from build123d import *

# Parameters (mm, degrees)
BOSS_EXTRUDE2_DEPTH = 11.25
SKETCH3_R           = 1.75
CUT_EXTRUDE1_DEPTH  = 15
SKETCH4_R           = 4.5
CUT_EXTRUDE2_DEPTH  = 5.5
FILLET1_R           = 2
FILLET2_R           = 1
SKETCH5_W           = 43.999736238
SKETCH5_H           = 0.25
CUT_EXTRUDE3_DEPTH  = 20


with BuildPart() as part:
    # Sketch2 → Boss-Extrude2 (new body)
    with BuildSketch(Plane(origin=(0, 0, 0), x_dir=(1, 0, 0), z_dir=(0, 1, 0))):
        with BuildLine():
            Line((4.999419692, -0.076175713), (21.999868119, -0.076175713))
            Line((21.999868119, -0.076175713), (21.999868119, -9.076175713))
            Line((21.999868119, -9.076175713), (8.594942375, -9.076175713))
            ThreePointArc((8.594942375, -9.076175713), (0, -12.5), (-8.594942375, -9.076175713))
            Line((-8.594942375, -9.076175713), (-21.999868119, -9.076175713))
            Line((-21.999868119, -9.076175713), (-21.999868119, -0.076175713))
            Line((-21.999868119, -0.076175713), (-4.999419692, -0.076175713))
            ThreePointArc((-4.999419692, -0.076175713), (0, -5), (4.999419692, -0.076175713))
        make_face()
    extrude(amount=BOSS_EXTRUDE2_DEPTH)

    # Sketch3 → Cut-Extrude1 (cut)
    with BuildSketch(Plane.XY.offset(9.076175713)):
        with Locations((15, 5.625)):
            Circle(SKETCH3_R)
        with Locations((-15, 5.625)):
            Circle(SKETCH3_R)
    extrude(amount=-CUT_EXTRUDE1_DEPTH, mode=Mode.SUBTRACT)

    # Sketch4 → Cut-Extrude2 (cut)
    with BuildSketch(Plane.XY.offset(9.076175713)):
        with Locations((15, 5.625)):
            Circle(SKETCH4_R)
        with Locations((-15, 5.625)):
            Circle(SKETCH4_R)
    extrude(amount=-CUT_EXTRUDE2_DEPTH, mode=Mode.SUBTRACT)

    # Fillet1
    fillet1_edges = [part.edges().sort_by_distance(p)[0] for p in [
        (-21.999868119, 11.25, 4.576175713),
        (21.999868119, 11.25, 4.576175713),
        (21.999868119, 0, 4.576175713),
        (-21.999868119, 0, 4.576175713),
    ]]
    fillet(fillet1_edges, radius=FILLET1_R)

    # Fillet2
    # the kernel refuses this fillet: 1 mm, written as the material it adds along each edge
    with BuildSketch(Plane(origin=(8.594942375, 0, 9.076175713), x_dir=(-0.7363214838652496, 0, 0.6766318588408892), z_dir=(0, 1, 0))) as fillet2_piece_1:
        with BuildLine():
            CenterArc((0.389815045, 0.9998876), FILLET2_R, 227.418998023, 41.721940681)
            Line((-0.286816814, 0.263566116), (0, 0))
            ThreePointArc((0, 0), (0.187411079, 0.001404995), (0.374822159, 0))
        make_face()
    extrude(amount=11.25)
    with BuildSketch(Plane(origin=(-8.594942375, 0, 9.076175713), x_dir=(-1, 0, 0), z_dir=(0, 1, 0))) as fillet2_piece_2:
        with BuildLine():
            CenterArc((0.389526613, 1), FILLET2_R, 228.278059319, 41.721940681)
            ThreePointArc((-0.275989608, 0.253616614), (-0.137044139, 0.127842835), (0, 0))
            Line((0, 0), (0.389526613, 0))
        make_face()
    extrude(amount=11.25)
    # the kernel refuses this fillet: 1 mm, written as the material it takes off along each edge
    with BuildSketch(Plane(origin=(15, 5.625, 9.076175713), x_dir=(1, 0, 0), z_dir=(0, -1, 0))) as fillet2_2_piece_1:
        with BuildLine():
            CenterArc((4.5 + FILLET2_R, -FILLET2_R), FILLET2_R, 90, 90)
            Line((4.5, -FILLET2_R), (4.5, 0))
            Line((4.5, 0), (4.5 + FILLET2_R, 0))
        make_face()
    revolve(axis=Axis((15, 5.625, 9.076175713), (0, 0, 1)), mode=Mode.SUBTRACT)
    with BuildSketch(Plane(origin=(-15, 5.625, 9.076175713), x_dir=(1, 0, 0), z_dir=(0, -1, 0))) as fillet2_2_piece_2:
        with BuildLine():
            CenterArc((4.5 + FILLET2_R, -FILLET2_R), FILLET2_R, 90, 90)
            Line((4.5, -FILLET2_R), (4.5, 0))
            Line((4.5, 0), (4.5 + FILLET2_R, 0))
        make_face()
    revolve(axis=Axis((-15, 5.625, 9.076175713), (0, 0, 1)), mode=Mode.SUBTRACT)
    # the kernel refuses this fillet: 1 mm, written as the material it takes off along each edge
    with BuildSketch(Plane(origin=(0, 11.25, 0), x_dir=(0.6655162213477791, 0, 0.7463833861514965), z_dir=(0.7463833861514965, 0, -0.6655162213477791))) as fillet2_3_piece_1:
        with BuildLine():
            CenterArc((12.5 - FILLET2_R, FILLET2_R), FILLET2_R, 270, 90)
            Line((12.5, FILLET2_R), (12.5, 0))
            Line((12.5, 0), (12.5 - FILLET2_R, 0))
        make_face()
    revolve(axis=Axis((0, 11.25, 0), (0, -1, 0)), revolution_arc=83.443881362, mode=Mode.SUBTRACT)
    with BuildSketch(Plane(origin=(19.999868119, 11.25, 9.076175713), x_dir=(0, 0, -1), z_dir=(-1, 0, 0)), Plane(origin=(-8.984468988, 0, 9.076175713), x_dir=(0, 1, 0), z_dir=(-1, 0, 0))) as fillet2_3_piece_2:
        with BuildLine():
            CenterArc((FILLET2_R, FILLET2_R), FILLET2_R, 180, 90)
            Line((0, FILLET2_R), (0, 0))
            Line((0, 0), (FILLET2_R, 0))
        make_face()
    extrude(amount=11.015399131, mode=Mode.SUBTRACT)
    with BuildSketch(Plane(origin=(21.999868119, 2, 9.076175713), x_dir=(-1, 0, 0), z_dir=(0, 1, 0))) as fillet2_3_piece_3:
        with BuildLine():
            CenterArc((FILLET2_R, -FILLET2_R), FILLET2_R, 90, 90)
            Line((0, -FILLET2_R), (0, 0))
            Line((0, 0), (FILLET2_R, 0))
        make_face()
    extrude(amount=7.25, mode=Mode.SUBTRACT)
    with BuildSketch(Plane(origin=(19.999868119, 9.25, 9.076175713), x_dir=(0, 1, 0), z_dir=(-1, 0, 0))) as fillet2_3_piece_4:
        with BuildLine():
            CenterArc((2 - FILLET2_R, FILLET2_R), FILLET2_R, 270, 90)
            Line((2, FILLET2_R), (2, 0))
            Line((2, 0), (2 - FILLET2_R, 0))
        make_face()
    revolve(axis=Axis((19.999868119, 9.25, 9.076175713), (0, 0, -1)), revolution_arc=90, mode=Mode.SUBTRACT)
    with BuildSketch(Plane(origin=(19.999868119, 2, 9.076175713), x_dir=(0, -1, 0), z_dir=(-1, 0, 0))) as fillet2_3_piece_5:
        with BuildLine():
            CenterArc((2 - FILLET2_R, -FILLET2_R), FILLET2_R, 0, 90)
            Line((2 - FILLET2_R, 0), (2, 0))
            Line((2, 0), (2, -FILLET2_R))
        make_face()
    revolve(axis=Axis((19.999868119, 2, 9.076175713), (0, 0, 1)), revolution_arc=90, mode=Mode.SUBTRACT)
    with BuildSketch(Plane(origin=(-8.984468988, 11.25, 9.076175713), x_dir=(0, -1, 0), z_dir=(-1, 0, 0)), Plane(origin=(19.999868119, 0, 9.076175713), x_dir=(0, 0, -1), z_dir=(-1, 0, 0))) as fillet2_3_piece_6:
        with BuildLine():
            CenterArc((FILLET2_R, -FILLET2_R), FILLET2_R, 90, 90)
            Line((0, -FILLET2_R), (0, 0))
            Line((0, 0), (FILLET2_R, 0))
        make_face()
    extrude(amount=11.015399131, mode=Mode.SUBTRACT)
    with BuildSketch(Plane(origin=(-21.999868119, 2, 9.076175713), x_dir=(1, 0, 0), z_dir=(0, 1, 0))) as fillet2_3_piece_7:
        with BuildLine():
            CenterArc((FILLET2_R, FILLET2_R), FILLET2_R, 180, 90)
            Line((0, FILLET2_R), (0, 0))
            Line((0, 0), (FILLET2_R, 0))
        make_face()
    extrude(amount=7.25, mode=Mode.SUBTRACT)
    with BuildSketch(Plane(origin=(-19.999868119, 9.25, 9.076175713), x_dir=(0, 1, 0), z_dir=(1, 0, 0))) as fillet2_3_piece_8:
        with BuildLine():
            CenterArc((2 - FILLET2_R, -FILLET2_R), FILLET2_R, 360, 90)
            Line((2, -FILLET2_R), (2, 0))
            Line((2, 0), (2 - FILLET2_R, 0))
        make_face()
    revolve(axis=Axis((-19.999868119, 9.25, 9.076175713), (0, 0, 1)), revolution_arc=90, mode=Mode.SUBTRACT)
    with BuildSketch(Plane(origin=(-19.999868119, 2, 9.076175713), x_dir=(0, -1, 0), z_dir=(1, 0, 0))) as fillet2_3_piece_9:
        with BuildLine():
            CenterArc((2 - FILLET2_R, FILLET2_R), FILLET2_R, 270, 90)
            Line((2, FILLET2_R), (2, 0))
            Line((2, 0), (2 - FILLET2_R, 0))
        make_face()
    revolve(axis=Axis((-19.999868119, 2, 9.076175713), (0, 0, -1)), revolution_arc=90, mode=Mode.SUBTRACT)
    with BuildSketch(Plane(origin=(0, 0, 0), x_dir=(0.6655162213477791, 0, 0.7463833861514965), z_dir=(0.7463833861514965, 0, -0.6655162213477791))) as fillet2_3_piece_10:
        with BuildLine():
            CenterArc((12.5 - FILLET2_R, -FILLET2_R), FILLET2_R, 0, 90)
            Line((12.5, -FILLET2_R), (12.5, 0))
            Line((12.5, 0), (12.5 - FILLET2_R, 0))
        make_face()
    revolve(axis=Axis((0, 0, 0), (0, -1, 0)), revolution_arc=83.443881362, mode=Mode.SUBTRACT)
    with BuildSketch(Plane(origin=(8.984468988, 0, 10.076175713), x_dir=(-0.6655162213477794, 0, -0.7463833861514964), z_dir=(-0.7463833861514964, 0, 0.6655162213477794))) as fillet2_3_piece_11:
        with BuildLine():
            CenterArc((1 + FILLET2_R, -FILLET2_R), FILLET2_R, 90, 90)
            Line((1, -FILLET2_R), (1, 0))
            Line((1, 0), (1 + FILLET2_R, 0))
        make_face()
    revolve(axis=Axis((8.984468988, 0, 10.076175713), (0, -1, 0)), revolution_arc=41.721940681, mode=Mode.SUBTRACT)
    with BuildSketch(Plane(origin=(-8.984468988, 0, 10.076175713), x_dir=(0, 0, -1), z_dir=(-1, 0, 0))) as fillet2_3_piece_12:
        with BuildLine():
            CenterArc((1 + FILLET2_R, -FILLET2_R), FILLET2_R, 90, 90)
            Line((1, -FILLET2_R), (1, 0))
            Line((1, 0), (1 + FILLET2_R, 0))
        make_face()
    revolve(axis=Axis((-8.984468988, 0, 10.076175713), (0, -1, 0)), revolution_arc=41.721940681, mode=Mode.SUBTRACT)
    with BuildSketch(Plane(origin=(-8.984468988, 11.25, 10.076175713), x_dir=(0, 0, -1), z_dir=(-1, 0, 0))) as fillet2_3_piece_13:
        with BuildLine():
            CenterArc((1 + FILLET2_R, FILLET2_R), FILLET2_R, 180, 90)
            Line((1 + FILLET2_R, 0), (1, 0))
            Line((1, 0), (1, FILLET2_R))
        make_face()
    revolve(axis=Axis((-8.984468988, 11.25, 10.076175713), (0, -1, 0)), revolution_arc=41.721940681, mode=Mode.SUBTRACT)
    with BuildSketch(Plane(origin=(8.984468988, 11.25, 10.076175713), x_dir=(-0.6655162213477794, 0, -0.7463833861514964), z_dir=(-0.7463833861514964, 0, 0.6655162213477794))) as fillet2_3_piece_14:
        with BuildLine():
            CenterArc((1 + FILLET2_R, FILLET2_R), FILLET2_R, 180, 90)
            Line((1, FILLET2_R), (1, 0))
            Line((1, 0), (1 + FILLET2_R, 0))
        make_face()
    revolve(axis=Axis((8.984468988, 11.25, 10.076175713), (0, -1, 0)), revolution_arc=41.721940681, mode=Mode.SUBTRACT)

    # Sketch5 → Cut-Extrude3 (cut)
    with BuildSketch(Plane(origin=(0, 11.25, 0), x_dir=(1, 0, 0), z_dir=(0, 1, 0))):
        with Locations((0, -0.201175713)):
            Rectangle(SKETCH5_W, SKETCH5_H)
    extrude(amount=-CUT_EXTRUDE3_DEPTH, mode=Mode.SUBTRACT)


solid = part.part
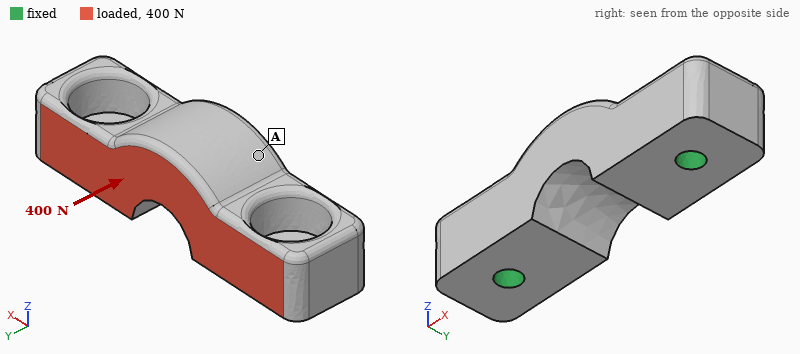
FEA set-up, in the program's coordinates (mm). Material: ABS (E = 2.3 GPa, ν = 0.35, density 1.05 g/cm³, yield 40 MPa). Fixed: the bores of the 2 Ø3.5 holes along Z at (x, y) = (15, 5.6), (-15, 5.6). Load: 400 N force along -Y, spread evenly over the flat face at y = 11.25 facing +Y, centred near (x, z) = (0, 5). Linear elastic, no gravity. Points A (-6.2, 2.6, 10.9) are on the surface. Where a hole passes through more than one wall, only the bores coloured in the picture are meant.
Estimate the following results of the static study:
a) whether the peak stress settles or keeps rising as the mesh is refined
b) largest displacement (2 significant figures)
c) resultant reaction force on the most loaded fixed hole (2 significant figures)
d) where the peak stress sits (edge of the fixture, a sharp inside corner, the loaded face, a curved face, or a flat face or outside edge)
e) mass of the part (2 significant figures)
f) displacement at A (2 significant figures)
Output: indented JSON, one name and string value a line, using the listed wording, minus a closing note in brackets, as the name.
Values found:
{
  "whether the peak stress settles or keeps rising as the mesh is refined": "keeps rising",
  "largest displacement": "0.20 mm",
  "resultant reaction force on the most loaded fixed hole": "200 N",
  "where the peak stress sits": "edge of the fixture",
  "mass of the part": "3.7 g",
  "displacement at A": "0.17 mm"
}
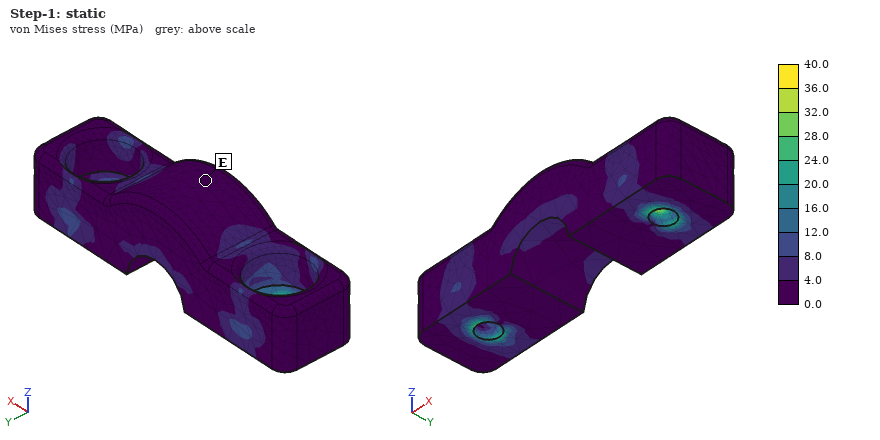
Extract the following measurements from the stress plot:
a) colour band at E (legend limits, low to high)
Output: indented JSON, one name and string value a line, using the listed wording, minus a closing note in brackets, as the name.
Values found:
{
  "colour band at E": "0.0 to 4.0 MPa"
}
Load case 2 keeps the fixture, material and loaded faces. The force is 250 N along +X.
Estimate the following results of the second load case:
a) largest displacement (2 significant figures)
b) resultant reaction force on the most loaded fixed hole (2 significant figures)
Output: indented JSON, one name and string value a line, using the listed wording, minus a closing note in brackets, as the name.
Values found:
{
  "largest displacement": "29 µm",
  "resultant reaction force on the most loaded fixed hole": "130 N"
}
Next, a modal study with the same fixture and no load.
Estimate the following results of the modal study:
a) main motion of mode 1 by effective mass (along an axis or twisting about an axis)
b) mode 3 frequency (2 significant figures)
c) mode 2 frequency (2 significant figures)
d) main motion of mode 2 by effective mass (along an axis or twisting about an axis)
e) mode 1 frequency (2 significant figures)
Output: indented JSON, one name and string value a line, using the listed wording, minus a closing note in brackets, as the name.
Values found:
{
  "main motion of mode 1 by effective mass": "along Y",
  "mode 3 frequency": "9200 Hz",
  "mode 2 frequency": "7700 Hz",
  "main motion of mode 2 by effective mass": "along Z",
  "mode 1 frequency": "4200 Hz"
}
